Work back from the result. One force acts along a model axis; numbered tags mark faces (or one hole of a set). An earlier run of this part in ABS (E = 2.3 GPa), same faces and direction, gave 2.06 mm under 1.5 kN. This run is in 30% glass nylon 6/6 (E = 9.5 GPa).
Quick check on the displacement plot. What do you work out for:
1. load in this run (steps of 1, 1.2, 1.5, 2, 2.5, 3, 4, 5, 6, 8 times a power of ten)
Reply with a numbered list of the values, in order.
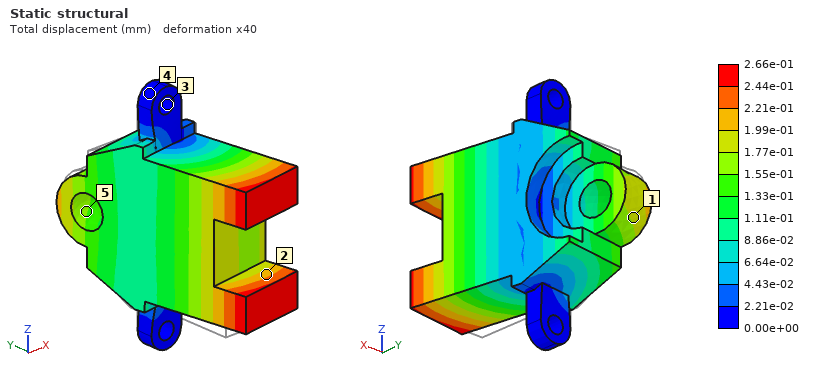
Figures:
1. 800 N
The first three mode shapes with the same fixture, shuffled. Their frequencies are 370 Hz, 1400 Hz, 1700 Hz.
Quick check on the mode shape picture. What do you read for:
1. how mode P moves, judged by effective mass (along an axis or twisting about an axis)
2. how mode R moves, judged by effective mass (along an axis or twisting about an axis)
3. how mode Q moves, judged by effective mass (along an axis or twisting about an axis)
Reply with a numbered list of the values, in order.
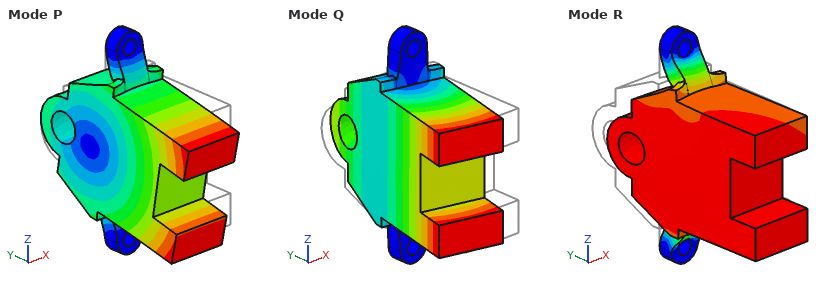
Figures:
1. along Z
2. along Y
3. along X
